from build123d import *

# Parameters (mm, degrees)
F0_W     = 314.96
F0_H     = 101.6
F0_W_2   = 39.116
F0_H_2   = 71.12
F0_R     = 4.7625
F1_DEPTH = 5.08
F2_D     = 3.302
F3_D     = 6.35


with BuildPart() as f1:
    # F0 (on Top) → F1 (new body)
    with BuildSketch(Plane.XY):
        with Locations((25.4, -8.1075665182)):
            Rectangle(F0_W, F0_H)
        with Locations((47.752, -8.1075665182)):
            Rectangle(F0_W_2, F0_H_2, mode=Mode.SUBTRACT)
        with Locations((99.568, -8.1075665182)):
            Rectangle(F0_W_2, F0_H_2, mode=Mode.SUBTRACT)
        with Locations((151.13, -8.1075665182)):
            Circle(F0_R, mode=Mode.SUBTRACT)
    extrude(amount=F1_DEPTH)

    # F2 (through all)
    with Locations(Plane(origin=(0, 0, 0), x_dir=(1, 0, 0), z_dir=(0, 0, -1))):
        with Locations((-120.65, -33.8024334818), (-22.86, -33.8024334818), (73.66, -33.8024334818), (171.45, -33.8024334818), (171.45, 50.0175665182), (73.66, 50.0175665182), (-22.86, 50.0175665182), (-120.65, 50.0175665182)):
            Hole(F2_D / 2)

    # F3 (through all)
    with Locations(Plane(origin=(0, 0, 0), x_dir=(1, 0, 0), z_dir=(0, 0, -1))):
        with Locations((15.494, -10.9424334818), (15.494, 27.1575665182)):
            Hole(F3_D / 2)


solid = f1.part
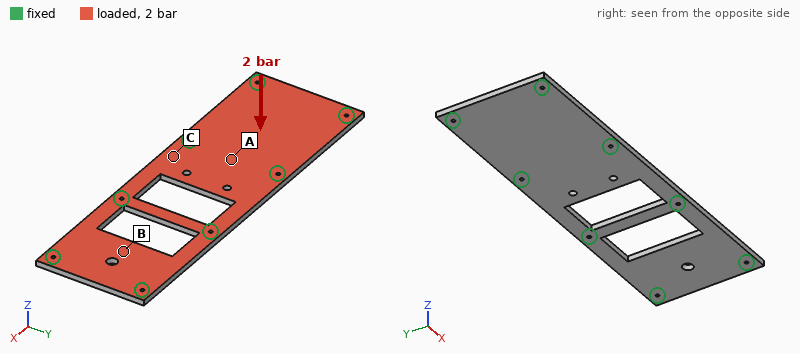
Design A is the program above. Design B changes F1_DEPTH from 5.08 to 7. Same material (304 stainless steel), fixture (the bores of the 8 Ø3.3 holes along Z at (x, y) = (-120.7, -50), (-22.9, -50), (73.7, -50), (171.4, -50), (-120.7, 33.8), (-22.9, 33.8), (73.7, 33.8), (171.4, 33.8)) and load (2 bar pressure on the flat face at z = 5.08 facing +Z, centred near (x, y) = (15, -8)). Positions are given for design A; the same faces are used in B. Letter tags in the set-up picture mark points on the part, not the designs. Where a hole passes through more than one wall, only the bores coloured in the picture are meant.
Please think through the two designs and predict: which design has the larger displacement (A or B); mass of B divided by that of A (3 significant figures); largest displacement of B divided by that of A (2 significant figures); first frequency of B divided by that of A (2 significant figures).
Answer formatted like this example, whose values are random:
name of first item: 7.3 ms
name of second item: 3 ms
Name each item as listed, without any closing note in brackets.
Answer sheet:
which design has the larger displacement: A
mass of B divided by that of A: 1.38
largest displacement of B divided by that of A: 0.41
first frequency of B divided by that of A: 1.3
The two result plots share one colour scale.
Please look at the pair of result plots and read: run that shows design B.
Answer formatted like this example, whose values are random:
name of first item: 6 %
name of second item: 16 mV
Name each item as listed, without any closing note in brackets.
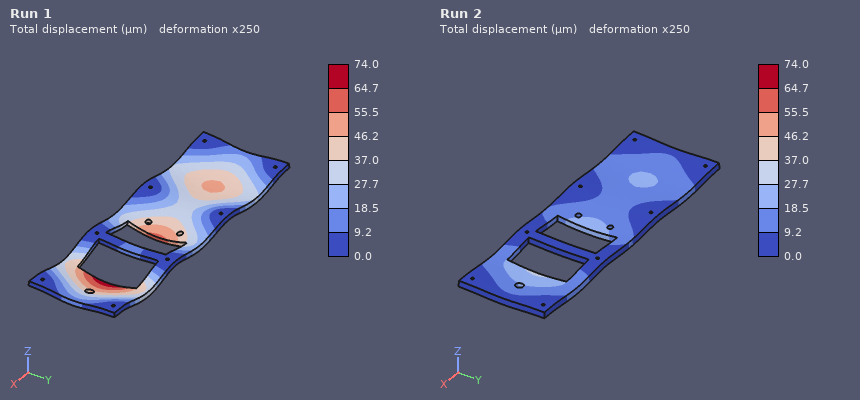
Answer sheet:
run that shows design B: Run 2
